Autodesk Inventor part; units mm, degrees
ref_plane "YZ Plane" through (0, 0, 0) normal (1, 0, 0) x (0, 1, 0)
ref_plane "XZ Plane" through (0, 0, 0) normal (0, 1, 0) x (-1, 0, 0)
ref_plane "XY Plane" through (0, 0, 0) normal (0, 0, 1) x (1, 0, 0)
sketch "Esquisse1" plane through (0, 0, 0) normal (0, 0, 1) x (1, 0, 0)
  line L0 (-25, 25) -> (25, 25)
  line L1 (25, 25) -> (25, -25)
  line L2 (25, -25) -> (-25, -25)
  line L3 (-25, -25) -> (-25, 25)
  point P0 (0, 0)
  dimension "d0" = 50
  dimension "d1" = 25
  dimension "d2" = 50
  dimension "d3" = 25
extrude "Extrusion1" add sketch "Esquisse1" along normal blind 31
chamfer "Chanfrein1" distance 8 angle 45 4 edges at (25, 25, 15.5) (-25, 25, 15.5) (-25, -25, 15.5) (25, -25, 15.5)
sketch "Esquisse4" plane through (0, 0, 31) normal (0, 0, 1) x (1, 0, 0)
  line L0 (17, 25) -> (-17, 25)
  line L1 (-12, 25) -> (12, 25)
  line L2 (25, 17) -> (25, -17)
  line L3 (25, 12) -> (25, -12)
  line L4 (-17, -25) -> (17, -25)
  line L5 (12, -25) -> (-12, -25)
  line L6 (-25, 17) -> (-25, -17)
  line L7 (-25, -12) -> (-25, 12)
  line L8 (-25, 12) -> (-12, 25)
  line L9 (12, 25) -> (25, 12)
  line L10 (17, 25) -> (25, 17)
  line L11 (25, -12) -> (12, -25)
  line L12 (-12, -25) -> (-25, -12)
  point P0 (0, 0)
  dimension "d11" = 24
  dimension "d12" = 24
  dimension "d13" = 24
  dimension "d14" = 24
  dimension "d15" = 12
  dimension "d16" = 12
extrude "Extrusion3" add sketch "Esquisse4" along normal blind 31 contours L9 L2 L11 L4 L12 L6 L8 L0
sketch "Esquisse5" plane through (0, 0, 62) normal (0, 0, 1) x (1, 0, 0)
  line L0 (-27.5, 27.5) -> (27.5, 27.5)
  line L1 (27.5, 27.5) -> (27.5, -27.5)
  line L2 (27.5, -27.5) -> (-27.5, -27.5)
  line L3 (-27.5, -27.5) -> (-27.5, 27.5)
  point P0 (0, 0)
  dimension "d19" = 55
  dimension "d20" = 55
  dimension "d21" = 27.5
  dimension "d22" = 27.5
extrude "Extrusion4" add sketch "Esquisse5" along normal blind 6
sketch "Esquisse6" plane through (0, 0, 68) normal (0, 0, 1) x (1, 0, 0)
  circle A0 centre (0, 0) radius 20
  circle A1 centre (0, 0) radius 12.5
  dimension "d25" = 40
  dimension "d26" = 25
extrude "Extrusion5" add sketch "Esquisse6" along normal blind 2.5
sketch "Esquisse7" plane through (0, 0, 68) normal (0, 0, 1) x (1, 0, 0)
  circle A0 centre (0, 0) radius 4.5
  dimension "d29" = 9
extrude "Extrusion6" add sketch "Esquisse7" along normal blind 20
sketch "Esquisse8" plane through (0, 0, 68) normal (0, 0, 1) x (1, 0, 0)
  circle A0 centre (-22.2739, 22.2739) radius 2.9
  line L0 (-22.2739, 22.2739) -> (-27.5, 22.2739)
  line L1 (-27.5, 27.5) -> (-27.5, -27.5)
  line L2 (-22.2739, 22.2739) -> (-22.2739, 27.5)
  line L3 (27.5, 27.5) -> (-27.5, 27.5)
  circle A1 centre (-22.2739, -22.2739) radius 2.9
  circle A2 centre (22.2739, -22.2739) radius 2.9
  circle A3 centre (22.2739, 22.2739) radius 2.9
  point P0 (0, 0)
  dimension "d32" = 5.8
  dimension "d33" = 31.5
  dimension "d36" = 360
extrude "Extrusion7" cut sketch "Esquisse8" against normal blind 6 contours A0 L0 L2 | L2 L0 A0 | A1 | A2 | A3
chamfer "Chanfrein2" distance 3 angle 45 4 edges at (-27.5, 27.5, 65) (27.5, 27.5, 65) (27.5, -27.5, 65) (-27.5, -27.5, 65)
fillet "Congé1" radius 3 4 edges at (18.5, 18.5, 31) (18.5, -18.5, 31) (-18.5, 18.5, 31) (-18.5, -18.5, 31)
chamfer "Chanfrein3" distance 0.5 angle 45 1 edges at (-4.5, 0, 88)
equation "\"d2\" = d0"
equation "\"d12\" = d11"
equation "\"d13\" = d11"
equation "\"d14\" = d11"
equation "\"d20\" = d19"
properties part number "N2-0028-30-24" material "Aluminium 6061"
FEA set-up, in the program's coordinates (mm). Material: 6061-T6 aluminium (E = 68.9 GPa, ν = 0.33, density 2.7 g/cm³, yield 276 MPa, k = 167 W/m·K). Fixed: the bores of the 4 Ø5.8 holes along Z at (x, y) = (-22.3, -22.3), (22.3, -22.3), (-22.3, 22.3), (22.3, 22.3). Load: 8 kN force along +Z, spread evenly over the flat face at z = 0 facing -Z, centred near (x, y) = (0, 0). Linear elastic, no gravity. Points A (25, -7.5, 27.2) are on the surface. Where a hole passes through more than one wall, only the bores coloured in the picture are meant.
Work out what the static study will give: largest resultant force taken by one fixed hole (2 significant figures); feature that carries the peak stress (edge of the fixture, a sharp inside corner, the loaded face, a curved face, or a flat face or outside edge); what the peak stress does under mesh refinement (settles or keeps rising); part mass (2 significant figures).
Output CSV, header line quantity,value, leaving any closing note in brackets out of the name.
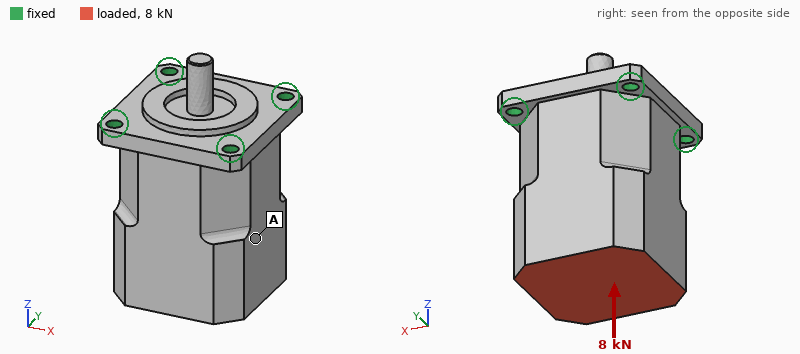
quantity,value
largest resultant force taken by one fixed hole,2.1 kN
feature that carries the peak stress,edge of the fixture
what the peak stress does under mesh refinement,keeps rising
part mass,440 g
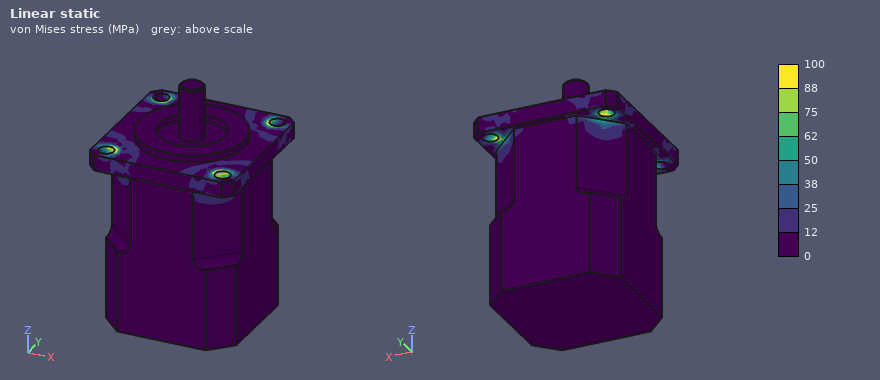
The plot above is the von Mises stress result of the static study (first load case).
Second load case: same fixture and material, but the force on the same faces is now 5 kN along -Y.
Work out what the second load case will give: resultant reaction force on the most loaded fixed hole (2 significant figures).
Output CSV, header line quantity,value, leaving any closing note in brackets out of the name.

quantity,value
resultant reaction force on the most loaded fixed hole,4.4 kN
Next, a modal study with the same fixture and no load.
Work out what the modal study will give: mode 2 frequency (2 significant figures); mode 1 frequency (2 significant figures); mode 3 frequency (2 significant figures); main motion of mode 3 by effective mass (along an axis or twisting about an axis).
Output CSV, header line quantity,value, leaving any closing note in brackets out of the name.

quantity,value
mode 2 frequency,3300 Hz
mode 1 frequency,3300 Hz
mode 3 frequency,6800 Hz
main motion of mode 3 by effective mass,along Z
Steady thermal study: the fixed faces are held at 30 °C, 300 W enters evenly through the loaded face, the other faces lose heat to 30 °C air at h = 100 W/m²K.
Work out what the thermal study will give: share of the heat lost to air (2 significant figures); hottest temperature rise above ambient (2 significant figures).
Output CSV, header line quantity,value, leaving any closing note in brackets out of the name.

quantity,value
share of the heat lost to air,22 %
hottest temperature rise above ambient,72 K
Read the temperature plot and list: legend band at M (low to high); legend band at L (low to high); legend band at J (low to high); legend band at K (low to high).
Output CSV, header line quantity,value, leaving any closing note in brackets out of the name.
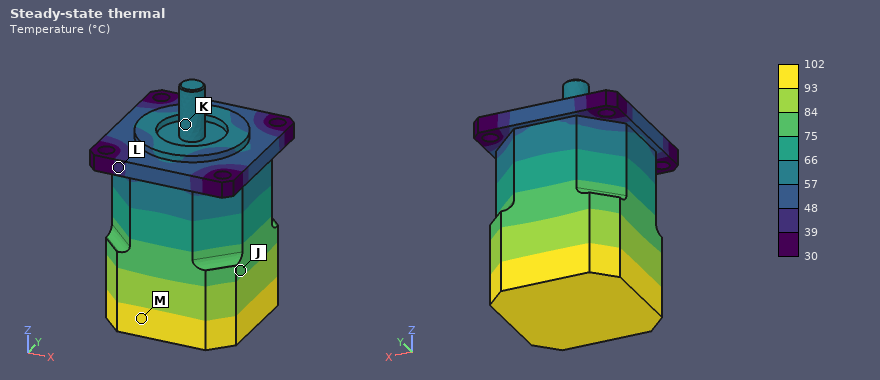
quantity,value
legend band at M,93 to 102 °C
legend band at L,39 to 48 °C
legend band at J,75 to 84 °C
legend band at K,57 to 66 °C
